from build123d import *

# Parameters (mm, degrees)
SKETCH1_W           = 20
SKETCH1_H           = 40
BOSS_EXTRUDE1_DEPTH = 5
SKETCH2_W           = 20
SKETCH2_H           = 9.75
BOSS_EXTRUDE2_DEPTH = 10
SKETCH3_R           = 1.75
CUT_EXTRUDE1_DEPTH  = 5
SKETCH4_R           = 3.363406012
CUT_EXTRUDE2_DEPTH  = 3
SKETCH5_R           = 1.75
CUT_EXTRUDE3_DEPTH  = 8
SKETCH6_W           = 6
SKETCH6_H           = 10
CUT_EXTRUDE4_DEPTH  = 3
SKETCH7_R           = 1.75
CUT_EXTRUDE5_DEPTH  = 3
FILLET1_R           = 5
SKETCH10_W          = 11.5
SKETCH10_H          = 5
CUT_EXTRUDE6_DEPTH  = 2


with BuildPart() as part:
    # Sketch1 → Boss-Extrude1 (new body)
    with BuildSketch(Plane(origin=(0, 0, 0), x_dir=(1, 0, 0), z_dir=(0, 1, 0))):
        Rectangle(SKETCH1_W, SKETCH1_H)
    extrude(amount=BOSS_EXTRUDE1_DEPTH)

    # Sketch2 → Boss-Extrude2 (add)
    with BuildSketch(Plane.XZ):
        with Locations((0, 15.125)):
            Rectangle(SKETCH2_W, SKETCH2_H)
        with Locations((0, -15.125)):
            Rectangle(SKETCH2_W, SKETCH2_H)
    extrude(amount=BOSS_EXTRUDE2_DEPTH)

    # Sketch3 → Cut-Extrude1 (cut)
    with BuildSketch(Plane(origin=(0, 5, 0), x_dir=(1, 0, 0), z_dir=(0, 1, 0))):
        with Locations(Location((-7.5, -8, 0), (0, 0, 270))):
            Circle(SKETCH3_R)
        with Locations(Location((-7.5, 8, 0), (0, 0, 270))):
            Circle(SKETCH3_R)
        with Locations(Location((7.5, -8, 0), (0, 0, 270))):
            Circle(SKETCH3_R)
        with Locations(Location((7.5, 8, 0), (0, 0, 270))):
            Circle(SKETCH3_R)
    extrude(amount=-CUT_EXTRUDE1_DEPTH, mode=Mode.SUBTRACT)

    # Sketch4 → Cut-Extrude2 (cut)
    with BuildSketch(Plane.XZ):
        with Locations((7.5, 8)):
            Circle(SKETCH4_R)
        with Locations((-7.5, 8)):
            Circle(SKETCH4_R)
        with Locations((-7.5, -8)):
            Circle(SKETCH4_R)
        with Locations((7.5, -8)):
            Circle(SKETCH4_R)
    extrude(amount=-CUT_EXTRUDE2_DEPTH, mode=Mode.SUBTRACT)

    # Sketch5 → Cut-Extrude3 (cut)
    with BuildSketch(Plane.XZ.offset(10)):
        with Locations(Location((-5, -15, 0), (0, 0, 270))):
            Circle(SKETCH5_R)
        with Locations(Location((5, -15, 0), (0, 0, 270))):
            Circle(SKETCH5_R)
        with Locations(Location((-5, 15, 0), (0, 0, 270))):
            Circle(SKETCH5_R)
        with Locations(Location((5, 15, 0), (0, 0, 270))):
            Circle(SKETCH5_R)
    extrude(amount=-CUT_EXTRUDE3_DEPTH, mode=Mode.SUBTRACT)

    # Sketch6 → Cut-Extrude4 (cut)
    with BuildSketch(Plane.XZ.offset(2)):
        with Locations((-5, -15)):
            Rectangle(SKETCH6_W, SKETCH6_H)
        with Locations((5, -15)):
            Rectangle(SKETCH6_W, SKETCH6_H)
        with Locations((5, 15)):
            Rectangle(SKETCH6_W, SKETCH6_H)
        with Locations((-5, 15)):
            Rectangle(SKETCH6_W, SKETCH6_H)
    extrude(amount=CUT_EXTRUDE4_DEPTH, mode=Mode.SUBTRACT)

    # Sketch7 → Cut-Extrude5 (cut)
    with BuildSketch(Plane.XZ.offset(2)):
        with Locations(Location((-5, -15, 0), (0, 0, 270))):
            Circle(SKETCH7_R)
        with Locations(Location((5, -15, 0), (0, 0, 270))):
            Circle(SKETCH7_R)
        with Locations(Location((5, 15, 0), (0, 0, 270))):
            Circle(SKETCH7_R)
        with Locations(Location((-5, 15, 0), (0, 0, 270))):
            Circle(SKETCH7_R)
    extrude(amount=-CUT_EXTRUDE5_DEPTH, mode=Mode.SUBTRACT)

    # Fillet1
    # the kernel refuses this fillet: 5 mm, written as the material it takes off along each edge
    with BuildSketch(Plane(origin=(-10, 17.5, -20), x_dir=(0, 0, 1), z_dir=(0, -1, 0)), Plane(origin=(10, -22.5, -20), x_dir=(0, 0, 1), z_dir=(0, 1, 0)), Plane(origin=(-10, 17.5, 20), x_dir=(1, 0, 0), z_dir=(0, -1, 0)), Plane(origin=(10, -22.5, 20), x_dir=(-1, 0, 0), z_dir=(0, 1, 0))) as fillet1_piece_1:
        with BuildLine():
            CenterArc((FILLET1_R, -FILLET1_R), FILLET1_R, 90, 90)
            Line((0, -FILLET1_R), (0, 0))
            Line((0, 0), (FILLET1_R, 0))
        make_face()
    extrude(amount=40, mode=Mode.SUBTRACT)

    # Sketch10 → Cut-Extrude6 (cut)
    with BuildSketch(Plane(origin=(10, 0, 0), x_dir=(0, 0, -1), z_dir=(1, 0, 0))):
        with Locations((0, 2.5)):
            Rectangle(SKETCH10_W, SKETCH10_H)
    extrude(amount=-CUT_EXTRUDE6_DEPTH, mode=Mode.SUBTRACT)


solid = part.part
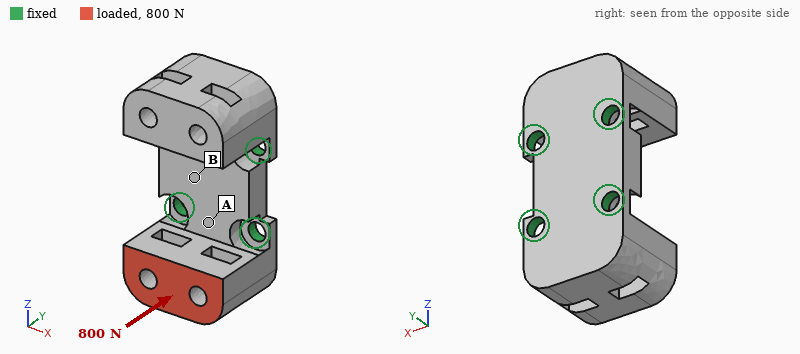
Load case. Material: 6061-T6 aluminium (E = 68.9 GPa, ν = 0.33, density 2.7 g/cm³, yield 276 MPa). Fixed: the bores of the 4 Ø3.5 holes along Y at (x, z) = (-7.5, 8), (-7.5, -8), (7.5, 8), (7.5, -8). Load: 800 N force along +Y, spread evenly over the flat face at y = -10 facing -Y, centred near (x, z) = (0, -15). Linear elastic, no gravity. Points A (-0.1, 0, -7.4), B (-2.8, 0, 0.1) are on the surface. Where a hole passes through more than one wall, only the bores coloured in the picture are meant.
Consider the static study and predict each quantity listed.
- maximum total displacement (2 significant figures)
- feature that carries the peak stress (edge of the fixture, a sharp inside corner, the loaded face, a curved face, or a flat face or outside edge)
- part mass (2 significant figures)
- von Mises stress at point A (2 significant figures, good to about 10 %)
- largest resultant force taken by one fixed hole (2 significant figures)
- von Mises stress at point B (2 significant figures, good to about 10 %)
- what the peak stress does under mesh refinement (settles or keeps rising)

52 µm
edge of the fixture
16 g
54 MPa
560 N
16 MPa
keeps rising
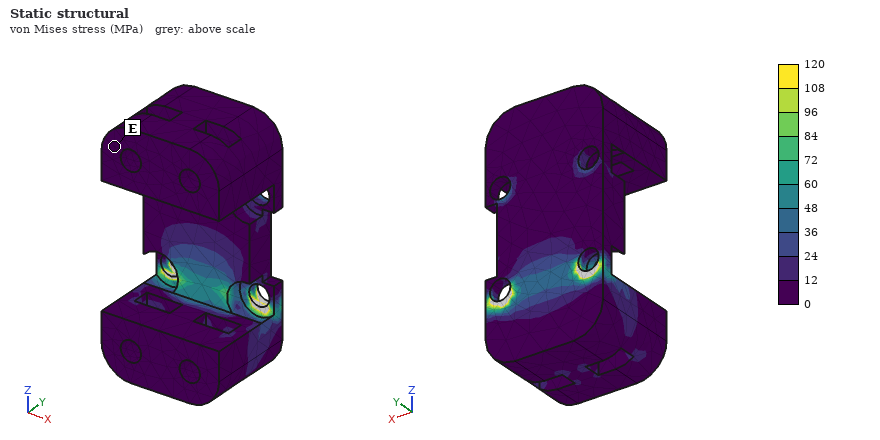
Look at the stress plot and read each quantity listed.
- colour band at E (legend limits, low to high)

0 to 12 MPa
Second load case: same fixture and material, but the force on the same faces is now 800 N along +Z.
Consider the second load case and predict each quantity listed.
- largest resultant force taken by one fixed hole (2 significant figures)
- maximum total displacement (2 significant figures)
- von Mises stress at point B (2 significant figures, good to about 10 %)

630 N
0.14 mm
37 MPa
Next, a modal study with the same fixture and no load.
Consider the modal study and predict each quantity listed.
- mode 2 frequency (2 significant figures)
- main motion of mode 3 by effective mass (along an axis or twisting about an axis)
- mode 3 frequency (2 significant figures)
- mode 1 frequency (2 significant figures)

8100 Hz
along X
16 kHz
7900 Hz
